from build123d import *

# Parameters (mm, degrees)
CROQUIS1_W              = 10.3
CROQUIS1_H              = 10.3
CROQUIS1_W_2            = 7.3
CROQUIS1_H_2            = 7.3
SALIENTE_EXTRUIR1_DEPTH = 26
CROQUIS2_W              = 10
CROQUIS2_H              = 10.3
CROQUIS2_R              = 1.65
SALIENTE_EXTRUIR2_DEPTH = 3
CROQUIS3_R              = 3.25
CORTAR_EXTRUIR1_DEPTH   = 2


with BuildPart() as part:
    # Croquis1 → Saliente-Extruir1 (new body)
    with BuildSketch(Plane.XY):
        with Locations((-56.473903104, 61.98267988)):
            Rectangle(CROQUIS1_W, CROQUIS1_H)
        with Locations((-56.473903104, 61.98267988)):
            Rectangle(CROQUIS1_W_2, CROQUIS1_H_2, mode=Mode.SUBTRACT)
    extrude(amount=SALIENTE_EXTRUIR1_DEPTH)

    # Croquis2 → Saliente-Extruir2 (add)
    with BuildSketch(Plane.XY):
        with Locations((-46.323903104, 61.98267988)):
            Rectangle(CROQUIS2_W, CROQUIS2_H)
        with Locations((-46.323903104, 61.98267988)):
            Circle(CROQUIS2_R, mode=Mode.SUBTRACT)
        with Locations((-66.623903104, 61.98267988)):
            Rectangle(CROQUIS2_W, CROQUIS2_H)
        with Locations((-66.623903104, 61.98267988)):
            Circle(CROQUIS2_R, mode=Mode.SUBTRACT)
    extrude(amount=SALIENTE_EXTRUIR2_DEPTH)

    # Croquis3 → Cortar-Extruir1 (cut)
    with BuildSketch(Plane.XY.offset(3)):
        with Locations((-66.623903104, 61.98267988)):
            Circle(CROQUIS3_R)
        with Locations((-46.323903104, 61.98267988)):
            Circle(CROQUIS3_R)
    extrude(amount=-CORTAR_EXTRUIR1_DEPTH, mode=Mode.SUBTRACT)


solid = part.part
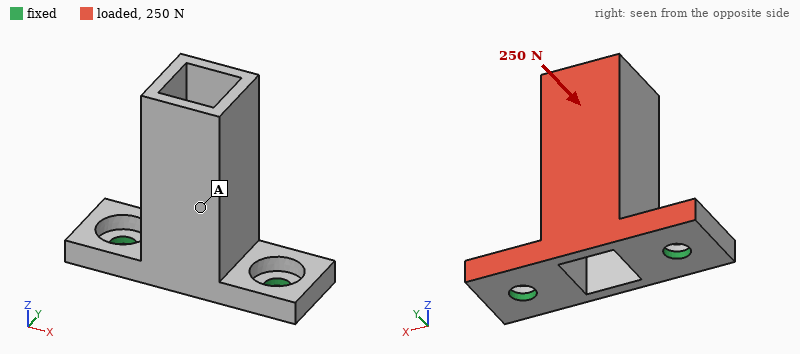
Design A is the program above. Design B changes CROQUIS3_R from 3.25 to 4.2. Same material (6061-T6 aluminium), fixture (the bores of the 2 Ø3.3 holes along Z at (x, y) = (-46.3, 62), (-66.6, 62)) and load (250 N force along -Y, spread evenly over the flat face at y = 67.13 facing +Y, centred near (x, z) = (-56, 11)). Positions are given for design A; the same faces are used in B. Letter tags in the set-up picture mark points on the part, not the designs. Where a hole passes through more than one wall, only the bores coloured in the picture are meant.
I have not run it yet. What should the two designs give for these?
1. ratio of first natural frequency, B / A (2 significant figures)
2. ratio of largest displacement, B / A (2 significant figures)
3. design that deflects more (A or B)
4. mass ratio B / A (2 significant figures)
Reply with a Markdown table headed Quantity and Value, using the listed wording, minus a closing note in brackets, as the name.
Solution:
| Quantity | Value |
|---|---|
| ratio of first natural frequency, B / A | 0.86 |
| ratio of largest displacement, B / A | 1.3 |
| design that deflects more | B |
| mass ratio B / A | 0.95 |
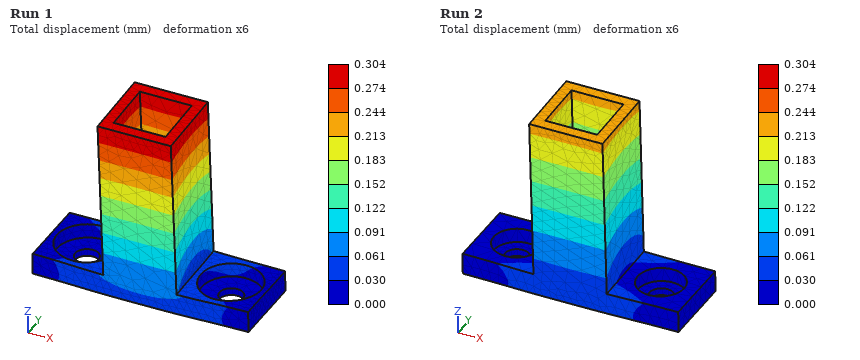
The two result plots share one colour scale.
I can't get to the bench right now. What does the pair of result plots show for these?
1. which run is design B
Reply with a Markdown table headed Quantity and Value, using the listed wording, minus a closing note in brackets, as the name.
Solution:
| Quantity | Value |
|---|---|
| which run is design B | Run 1 |
